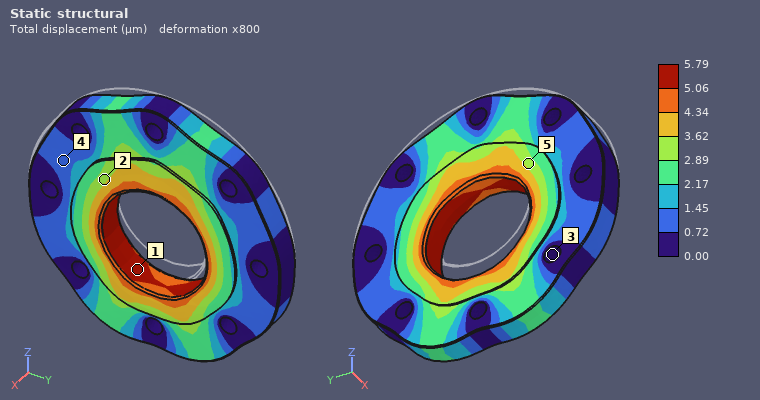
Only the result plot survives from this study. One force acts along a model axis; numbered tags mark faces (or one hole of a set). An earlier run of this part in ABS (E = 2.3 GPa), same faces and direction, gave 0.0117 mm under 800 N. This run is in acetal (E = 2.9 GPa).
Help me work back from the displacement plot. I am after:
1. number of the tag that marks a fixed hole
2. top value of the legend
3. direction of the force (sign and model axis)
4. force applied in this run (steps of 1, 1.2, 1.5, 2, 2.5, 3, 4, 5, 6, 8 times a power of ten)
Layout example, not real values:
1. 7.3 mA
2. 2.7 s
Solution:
1. 3
2. 5.79 µm
3. -Z
4. 500 N
